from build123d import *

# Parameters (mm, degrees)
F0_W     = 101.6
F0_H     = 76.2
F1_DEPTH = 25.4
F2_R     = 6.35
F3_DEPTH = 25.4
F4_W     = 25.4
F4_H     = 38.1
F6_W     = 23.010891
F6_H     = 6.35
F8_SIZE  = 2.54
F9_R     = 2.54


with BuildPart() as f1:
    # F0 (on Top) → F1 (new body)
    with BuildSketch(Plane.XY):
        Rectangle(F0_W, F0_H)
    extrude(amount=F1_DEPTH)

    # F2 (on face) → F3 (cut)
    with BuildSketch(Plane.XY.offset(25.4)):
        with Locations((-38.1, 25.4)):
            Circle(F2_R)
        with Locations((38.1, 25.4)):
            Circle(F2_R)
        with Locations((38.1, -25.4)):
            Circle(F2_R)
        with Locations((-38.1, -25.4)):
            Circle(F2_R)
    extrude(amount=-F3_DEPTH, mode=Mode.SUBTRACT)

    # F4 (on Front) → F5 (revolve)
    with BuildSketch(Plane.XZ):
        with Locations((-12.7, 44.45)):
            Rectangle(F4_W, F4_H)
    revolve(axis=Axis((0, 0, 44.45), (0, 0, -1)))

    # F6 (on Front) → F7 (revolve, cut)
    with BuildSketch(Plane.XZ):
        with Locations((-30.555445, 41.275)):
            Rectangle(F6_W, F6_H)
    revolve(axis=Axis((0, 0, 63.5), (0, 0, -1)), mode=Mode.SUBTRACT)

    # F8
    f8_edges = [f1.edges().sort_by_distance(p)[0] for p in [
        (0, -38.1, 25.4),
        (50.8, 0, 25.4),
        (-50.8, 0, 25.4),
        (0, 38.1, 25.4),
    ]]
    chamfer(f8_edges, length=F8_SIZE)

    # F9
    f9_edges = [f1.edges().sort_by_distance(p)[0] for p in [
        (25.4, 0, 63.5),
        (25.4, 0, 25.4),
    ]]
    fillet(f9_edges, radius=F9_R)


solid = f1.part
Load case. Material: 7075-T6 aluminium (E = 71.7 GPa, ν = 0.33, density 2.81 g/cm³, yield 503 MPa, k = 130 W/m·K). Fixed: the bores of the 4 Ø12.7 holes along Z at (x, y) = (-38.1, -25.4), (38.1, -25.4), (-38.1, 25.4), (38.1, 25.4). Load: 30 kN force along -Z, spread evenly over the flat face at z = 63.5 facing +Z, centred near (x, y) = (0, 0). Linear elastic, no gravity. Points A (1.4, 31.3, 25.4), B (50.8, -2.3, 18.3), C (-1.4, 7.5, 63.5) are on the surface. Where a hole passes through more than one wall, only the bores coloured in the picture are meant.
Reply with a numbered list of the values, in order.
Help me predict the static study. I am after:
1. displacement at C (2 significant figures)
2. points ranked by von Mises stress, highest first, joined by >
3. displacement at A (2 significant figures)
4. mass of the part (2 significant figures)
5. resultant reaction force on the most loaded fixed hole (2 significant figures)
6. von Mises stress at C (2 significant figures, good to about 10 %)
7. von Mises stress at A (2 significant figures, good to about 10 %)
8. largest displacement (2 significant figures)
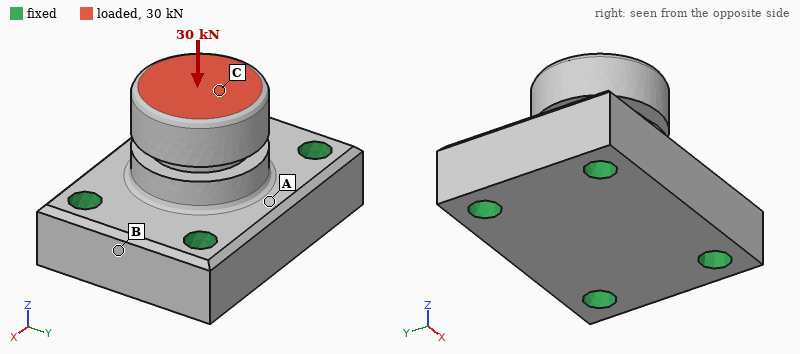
1. 23 µm
2. C > A > B
3. 10 µm
4. 710 g
5. 7.8 kN
6. 21 MPa
7. 12 MPa
8. 23 µm
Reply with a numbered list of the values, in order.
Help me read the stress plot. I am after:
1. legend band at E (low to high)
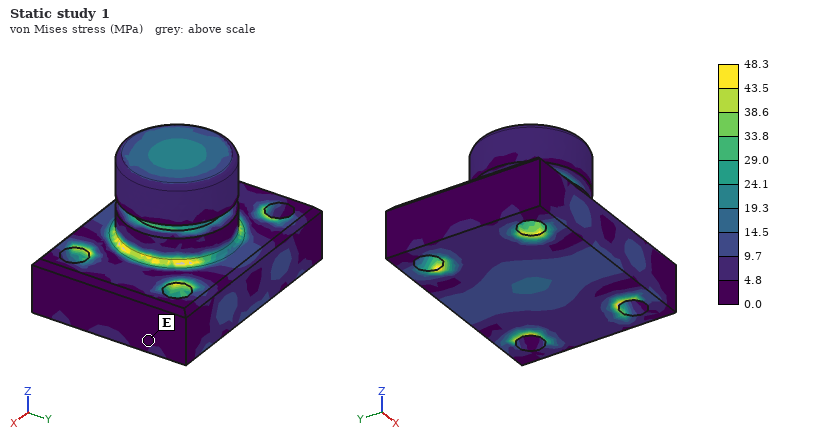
1. 0.0 to 4.8 MPa
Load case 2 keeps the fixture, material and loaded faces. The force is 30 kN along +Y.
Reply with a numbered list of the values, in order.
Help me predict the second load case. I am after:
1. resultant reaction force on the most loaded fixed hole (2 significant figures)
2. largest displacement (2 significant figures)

1. 17 kN
2. 0.15 mm
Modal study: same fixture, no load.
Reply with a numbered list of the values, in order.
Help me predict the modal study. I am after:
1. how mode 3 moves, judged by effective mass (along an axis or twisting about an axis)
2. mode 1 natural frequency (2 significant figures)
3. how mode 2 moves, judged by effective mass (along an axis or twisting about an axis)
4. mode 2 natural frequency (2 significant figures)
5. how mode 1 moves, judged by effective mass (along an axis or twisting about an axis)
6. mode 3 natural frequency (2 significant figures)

1. along Z
2. 8000 Hz
3. along X
4. 9400 Hz
5. along Y
6. 12 kHz
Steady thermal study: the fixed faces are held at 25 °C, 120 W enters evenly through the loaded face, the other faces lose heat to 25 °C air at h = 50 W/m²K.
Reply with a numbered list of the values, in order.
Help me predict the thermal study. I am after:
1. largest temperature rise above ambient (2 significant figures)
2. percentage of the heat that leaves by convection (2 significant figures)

1. 31 K
2. 7.9 %
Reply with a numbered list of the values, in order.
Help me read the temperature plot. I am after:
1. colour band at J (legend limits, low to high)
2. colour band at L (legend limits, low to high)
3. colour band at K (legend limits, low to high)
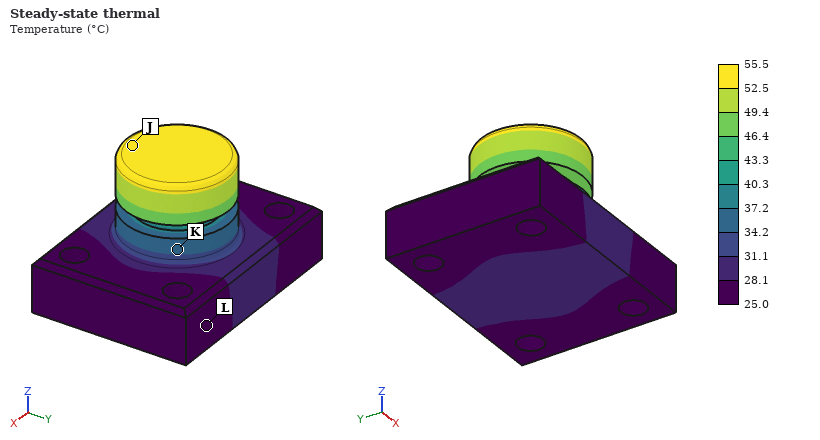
1. 52.5 to 55.5 °C
2. 25.0 to 28.1 °C
3. 34.2 to 37.2 °C
